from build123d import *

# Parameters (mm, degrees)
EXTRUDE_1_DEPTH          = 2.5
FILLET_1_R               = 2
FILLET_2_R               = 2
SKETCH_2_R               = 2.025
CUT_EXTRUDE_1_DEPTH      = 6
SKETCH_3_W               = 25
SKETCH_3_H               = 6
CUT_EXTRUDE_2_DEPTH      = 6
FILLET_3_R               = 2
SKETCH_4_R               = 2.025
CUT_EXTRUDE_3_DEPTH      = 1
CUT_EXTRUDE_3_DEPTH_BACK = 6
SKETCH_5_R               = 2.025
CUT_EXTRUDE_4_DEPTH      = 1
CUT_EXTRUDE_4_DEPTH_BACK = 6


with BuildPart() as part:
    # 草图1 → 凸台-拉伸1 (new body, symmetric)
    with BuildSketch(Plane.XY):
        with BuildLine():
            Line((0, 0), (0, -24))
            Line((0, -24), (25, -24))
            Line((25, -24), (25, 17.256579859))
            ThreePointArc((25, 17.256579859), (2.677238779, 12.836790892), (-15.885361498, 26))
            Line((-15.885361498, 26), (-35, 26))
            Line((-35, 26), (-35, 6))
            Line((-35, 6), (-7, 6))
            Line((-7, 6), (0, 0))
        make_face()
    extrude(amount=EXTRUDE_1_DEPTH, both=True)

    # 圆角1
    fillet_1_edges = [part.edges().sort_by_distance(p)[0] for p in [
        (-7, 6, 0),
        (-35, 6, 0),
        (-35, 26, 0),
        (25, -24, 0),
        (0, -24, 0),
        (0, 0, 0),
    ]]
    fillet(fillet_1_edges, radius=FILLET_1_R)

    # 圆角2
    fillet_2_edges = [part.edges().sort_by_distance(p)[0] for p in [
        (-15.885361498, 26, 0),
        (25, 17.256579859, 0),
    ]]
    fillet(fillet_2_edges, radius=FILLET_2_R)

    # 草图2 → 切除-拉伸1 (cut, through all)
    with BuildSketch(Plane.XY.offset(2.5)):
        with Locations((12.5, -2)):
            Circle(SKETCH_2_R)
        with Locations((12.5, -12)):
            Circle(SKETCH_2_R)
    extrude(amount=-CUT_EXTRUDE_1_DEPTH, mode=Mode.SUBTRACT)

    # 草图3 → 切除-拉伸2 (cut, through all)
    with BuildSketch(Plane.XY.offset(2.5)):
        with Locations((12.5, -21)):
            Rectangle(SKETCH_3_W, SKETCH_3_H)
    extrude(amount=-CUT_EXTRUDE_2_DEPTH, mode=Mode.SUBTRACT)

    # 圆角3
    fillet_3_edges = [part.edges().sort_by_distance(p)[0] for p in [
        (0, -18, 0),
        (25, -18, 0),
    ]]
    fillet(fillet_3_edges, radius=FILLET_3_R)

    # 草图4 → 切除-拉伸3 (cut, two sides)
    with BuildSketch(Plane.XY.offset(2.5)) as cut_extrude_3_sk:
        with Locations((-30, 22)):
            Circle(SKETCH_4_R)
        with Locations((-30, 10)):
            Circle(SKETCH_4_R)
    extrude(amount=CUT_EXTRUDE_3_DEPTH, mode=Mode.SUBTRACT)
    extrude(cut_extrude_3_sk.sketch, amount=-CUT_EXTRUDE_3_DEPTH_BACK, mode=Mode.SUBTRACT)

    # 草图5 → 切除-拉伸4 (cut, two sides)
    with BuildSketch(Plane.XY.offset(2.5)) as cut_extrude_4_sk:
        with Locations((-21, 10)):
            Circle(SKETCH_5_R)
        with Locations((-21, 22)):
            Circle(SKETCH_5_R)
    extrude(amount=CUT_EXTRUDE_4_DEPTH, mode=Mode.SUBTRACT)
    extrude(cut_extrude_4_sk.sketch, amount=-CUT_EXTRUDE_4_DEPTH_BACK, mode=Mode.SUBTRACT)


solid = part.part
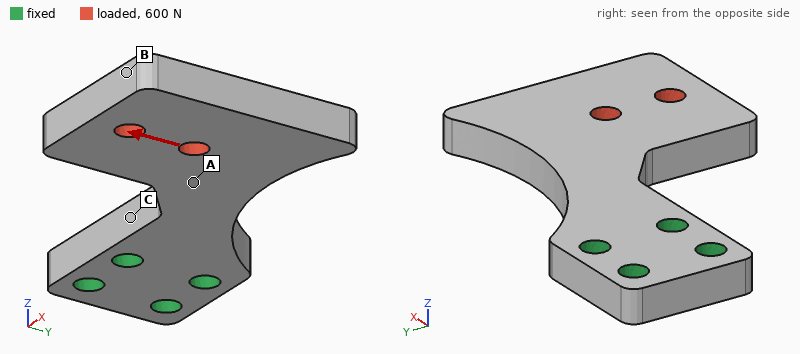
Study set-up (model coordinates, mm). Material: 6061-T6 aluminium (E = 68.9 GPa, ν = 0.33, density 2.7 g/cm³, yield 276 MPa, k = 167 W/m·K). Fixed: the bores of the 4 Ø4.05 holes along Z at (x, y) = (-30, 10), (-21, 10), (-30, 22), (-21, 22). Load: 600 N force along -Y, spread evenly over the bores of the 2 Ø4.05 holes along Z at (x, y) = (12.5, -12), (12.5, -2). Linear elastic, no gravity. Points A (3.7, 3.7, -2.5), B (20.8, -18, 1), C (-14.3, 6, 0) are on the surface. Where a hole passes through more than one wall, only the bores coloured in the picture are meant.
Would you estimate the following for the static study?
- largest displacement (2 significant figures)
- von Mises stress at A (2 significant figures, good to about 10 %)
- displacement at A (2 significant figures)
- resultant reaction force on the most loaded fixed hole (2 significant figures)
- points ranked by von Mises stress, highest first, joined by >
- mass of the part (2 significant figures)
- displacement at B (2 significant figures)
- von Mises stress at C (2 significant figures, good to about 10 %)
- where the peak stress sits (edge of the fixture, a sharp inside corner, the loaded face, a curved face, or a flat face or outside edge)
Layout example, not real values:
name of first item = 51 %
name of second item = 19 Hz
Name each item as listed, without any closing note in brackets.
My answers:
largest displacement = 0.26 mm
von Mises stress at A = 27 MPa
displacement at A = 0.082 mm
resultant reaction force on the most loaded fixed hole = 1.5 kN
points ranked by von Mises stress, highest first, joined by > = C > A > B
mass of the part = 18 g
displacement at B = 0.25 mm
von Mises stress at C = 88 MPa
where the peak stress sits = a curved face
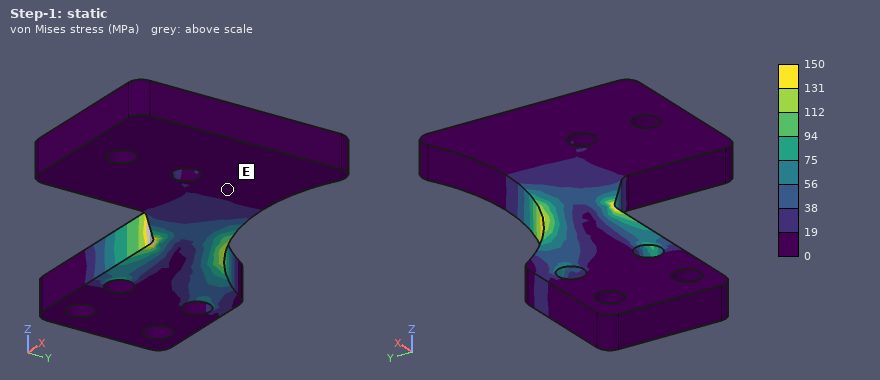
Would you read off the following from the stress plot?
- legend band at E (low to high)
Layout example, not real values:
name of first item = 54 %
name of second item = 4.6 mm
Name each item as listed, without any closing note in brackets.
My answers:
legend band at E = 0 to 19 MPa
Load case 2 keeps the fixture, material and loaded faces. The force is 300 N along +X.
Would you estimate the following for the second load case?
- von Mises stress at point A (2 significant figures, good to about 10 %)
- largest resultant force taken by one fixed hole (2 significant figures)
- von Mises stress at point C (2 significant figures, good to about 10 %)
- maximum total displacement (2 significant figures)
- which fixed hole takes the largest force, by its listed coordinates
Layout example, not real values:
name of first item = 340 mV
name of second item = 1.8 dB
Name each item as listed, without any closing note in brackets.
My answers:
von Mises stress at point A = 15 MPa
largest resultant force taken by one fixed hole = 650 N
von Mises stress at point C = 38 MPa
maximum total displacement = 0.12 mm
which fixed hole takes the largest force, by its listed coordinates = (-21, 10)
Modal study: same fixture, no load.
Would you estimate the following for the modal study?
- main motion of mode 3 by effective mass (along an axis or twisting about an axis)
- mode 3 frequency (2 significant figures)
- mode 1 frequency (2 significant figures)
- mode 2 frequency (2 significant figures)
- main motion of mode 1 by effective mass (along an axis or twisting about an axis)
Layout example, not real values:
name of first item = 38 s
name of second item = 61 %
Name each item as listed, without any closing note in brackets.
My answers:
main motion of mode 3 by effective mass = twisting about X
mode 3 frequency = 3300 Hz
mode 1 frequency = 1200 Hz
mode 2 frequency = 2600 Hz
main motion of mode 1 by effective mass = along Z
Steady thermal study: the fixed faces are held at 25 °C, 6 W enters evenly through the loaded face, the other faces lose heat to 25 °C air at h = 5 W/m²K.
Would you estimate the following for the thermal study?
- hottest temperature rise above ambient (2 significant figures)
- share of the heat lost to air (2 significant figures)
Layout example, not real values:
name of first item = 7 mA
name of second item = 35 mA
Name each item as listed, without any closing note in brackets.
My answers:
hottest temperature rise above ambient = 20 K
share of the heat lost to air = 3.3 %
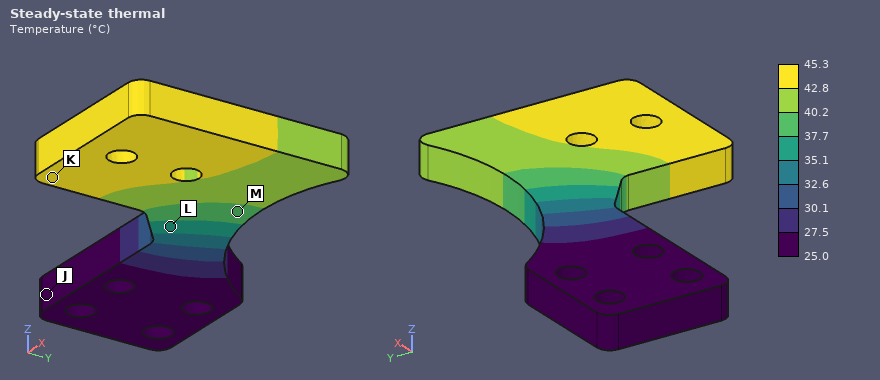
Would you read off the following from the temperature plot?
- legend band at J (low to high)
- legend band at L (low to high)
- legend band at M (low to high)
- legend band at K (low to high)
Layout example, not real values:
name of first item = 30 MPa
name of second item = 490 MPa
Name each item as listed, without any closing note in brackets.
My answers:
legend band at J = 25.0 to 27.5 °C
legend band at L = 35.1 to 37.7 °C
legend band at M = 37.7 to 40.2 °C
legend band at K = 42.8 to 45.3 °C
